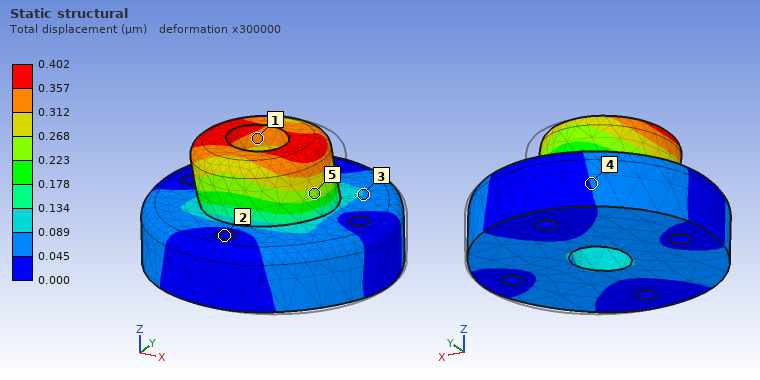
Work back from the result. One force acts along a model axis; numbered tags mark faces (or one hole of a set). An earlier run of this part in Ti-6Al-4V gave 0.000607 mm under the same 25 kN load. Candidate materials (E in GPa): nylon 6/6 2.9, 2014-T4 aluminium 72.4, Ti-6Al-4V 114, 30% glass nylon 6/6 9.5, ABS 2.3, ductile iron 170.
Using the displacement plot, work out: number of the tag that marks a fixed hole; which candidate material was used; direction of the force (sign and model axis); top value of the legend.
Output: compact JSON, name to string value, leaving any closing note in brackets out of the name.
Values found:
{"number of the tag that marks a fixed hole": "2", "which candidate material was used": "ductile iron", "direction of the force": "-X", "top value of the legend": "0.402 µm"}
